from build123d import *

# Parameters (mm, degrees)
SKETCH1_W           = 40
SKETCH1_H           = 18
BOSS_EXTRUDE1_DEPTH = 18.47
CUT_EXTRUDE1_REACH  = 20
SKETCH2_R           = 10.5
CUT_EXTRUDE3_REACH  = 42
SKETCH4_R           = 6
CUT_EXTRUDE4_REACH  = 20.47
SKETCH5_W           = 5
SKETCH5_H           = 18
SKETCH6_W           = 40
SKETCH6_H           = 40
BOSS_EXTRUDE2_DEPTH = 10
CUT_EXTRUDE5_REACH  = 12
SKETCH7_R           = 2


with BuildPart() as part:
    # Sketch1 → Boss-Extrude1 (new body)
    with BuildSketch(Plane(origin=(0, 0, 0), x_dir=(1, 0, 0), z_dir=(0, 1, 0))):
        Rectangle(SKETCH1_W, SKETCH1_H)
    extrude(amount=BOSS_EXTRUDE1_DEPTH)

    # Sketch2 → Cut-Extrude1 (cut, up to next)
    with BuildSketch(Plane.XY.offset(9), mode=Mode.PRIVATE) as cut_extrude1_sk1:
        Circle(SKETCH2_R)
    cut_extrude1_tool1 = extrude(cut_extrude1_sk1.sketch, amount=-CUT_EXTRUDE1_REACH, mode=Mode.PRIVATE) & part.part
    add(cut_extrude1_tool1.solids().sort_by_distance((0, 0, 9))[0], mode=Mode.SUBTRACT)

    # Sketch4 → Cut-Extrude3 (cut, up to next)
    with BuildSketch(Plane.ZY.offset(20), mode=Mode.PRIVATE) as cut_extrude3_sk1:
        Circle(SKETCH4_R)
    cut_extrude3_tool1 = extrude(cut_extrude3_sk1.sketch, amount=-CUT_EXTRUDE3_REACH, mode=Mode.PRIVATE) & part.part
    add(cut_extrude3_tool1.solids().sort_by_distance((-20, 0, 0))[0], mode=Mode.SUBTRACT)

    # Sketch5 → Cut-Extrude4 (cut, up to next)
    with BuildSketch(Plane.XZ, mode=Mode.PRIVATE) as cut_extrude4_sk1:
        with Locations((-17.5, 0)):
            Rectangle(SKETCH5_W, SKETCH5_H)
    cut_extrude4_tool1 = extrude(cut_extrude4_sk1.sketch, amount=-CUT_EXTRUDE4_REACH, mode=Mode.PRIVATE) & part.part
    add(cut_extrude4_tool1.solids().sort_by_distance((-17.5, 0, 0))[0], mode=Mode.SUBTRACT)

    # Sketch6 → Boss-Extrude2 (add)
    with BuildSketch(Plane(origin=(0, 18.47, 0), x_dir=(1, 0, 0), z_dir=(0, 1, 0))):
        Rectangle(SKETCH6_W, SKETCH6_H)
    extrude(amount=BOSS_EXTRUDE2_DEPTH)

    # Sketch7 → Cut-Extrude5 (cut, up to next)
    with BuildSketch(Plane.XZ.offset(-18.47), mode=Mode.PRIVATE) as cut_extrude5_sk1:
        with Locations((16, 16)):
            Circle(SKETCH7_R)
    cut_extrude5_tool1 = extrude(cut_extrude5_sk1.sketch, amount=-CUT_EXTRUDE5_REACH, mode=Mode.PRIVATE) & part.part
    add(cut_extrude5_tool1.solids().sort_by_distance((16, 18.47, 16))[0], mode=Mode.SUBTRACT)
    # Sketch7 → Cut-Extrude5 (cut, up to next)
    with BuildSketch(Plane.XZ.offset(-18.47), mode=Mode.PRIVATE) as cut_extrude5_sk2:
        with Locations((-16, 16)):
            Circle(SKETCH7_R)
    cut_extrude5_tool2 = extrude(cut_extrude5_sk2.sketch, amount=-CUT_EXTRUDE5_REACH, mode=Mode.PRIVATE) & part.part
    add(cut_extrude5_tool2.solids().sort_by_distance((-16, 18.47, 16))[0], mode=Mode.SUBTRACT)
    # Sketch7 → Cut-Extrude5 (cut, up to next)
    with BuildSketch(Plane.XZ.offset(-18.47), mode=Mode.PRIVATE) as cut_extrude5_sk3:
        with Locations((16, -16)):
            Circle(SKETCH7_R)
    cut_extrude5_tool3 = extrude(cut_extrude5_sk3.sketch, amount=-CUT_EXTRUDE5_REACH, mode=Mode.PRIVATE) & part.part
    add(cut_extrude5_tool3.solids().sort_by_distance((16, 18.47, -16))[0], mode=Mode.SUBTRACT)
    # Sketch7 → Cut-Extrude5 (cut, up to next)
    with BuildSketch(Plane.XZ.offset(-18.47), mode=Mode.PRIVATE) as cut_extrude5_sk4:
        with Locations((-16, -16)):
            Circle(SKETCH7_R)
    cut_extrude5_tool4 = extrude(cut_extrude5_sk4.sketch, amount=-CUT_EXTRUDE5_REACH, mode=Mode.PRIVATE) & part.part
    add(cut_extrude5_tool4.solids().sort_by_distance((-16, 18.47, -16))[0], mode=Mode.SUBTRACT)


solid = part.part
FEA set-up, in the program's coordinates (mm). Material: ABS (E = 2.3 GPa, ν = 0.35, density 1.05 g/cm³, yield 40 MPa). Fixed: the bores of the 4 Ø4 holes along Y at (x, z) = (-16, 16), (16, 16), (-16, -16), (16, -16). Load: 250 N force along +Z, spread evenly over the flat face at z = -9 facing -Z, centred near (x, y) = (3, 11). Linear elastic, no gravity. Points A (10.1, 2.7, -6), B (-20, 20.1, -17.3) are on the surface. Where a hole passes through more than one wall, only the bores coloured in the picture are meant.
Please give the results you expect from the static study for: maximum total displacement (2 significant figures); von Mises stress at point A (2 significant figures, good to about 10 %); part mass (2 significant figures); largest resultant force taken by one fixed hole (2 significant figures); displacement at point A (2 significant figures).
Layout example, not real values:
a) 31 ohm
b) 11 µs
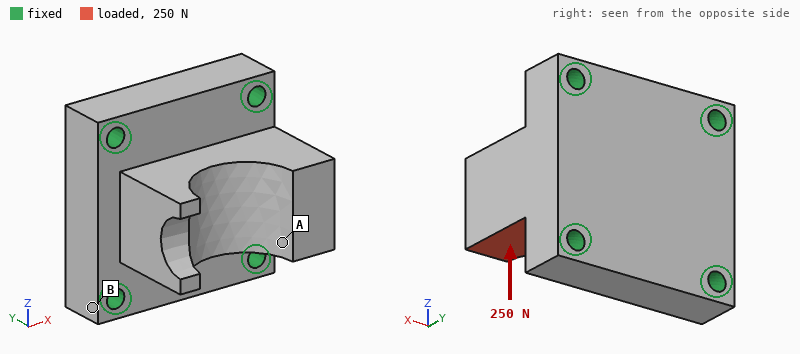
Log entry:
a) 37 µm
b) 0.56 MPa
c) 25 g
d) 98 N
e) 25 µm
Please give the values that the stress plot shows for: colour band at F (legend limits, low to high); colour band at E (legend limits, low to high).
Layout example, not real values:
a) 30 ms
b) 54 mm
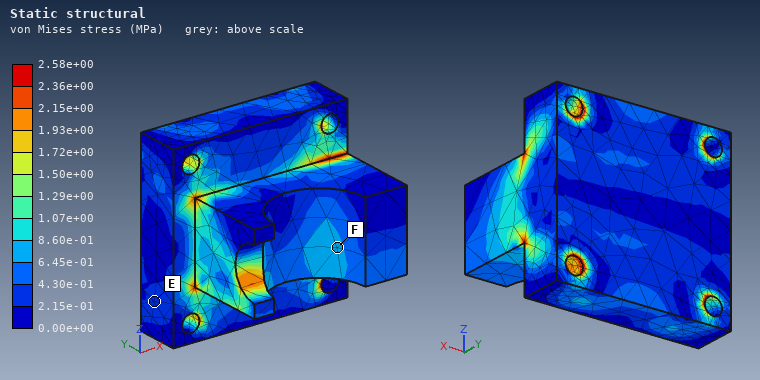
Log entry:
a) 6.45e-01 to 8.60e-01 MPa
b) 2.15e-01 to 4.30e-01 MPa
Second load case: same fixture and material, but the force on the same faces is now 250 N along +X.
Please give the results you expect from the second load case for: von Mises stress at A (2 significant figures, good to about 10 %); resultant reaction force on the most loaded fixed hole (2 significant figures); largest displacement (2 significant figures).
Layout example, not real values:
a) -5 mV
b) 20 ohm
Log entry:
a) 0.87 MPa
b) 98 N
c) 51 µm
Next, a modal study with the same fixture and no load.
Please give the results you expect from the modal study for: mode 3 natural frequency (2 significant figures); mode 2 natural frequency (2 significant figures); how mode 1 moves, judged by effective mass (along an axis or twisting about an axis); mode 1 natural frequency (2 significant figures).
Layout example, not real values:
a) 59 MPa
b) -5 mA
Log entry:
a) 6200 Hz
b) 6200 Hz
c) along X
d) 5600 Hz
